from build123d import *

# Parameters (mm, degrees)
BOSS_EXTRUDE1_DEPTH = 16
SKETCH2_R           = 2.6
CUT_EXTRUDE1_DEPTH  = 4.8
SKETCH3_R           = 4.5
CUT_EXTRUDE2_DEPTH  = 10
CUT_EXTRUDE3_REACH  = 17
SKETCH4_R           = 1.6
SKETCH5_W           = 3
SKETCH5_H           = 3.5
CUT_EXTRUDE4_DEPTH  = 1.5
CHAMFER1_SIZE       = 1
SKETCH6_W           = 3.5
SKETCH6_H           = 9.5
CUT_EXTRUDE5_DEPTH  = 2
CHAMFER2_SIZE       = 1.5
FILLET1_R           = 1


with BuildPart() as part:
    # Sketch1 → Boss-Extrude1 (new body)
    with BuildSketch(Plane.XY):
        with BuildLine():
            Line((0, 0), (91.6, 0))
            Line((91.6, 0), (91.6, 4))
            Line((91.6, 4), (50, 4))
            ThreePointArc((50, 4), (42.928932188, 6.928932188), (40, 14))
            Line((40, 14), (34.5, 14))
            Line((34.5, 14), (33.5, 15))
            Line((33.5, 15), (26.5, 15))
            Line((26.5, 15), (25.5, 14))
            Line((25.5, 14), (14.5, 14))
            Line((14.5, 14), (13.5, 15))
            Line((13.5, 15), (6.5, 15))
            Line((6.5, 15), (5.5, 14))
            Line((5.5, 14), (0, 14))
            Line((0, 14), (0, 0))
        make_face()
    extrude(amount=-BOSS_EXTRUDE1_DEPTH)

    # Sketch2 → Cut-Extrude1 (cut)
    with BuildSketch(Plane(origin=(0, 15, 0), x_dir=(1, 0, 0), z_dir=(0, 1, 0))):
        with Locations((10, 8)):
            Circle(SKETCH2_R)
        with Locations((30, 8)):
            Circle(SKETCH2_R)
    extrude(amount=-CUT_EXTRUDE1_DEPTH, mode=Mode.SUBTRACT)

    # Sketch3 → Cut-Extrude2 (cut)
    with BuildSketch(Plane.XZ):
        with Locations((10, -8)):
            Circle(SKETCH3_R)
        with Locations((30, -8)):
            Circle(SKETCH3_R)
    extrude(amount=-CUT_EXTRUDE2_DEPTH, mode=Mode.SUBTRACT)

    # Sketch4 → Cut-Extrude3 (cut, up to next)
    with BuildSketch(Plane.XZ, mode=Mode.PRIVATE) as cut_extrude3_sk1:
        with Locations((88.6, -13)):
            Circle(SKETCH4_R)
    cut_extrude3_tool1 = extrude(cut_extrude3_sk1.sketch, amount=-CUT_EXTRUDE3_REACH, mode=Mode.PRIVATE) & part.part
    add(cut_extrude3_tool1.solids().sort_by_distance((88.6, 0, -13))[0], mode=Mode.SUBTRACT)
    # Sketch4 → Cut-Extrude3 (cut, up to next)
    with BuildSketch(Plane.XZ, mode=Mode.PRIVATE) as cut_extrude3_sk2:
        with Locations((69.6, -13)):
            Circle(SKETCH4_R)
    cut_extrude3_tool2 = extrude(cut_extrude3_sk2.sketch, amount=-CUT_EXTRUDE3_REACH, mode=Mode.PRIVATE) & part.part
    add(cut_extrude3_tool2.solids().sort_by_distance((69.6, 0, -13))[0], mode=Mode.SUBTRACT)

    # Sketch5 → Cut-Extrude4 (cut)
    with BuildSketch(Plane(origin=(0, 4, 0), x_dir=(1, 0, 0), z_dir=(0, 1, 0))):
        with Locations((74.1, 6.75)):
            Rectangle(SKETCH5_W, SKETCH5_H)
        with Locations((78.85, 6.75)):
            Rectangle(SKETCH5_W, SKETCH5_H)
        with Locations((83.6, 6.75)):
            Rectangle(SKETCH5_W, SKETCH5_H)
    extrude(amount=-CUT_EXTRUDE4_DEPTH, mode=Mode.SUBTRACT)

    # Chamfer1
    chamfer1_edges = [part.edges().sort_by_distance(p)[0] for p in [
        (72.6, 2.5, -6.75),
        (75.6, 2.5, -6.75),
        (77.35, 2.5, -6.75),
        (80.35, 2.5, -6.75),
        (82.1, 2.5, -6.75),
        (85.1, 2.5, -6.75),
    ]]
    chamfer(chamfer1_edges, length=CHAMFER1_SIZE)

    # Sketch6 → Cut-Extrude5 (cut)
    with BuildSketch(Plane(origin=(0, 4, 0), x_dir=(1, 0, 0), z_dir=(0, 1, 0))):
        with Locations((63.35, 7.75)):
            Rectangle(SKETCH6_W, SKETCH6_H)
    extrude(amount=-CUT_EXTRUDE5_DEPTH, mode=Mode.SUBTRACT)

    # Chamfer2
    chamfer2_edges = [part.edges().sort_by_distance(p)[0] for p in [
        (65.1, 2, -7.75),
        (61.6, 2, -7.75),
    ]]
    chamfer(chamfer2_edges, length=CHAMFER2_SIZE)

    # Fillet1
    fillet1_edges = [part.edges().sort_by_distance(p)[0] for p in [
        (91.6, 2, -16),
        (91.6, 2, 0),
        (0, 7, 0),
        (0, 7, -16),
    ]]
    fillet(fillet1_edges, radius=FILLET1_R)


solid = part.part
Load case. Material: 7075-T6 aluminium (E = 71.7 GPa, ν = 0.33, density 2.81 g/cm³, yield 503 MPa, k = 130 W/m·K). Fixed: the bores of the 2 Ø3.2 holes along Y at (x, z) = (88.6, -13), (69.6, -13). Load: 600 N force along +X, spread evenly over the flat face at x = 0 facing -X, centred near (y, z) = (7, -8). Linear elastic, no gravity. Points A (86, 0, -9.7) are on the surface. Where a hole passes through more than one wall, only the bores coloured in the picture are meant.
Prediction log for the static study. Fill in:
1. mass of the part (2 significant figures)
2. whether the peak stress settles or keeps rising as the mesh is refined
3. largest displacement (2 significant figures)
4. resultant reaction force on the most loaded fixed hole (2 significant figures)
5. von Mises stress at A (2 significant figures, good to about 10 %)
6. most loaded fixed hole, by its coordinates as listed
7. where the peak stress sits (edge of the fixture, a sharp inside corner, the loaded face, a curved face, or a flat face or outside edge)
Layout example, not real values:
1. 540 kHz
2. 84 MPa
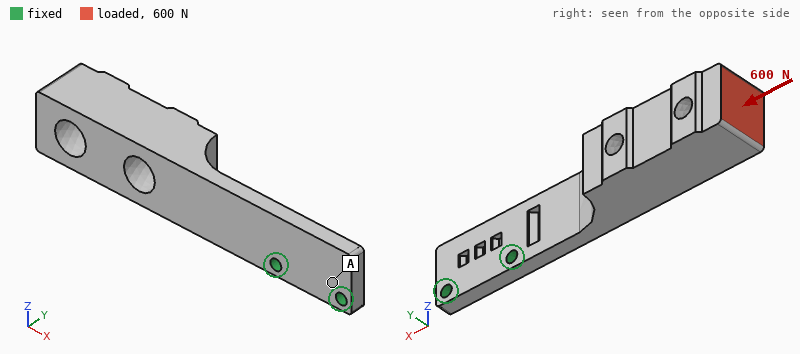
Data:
1. 32 g
2. keeps rising
3. 0.88 mm
4. 480 N
5. 17 MPa
6. (69.6, -13)
7. edge of the fixture
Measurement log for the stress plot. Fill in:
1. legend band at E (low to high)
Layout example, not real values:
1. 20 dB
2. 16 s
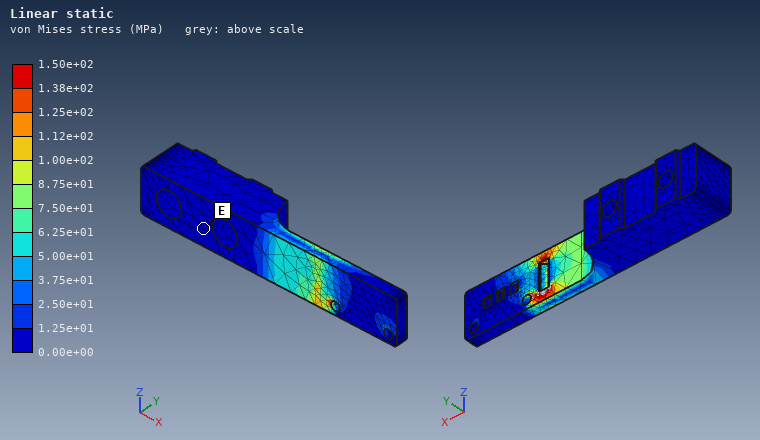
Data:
1. 0.00e+00 to 1.25e+01 MPa
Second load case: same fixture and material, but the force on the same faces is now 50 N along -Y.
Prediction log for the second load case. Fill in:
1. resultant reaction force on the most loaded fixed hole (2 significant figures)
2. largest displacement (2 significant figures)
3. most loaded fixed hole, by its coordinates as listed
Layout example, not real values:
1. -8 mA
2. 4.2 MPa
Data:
1. 110 N
2. 0.86 mm
3. (69.6, -13)
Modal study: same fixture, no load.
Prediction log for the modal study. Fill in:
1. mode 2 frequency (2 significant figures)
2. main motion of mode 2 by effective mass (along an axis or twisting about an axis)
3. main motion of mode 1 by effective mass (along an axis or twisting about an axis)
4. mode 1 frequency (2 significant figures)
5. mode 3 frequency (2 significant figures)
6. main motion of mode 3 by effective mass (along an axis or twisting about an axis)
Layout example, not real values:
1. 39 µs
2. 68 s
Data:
1. 1200 Hz
2. along Z
3. along Y
4. 370 Hz
5. 2700 Hz
6. twisting about X
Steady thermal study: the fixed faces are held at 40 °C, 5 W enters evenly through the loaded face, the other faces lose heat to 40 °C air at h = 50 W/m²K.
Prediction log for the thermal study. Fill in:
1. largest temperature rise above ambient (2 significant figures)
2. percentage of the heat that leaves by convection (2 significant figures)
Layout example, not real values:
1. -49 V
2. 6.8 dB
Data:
1. 17 K
2. 50 %
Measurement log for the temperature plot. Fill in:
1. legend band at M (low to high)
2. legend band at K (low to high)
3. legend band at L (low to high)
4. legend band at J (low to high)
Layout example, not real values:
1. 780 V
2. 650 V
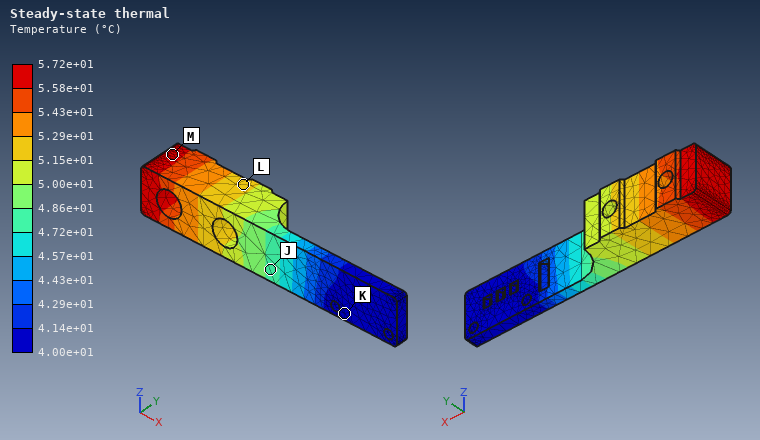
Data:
1. 5.58e+01 to 5.72e+01 °C
2. 4.00e+01 to 4.14e+01 °C
3. 5.15e+01 to 5.29e+01 °C
4. 4.72e+01 to 4.86e+01 °C
